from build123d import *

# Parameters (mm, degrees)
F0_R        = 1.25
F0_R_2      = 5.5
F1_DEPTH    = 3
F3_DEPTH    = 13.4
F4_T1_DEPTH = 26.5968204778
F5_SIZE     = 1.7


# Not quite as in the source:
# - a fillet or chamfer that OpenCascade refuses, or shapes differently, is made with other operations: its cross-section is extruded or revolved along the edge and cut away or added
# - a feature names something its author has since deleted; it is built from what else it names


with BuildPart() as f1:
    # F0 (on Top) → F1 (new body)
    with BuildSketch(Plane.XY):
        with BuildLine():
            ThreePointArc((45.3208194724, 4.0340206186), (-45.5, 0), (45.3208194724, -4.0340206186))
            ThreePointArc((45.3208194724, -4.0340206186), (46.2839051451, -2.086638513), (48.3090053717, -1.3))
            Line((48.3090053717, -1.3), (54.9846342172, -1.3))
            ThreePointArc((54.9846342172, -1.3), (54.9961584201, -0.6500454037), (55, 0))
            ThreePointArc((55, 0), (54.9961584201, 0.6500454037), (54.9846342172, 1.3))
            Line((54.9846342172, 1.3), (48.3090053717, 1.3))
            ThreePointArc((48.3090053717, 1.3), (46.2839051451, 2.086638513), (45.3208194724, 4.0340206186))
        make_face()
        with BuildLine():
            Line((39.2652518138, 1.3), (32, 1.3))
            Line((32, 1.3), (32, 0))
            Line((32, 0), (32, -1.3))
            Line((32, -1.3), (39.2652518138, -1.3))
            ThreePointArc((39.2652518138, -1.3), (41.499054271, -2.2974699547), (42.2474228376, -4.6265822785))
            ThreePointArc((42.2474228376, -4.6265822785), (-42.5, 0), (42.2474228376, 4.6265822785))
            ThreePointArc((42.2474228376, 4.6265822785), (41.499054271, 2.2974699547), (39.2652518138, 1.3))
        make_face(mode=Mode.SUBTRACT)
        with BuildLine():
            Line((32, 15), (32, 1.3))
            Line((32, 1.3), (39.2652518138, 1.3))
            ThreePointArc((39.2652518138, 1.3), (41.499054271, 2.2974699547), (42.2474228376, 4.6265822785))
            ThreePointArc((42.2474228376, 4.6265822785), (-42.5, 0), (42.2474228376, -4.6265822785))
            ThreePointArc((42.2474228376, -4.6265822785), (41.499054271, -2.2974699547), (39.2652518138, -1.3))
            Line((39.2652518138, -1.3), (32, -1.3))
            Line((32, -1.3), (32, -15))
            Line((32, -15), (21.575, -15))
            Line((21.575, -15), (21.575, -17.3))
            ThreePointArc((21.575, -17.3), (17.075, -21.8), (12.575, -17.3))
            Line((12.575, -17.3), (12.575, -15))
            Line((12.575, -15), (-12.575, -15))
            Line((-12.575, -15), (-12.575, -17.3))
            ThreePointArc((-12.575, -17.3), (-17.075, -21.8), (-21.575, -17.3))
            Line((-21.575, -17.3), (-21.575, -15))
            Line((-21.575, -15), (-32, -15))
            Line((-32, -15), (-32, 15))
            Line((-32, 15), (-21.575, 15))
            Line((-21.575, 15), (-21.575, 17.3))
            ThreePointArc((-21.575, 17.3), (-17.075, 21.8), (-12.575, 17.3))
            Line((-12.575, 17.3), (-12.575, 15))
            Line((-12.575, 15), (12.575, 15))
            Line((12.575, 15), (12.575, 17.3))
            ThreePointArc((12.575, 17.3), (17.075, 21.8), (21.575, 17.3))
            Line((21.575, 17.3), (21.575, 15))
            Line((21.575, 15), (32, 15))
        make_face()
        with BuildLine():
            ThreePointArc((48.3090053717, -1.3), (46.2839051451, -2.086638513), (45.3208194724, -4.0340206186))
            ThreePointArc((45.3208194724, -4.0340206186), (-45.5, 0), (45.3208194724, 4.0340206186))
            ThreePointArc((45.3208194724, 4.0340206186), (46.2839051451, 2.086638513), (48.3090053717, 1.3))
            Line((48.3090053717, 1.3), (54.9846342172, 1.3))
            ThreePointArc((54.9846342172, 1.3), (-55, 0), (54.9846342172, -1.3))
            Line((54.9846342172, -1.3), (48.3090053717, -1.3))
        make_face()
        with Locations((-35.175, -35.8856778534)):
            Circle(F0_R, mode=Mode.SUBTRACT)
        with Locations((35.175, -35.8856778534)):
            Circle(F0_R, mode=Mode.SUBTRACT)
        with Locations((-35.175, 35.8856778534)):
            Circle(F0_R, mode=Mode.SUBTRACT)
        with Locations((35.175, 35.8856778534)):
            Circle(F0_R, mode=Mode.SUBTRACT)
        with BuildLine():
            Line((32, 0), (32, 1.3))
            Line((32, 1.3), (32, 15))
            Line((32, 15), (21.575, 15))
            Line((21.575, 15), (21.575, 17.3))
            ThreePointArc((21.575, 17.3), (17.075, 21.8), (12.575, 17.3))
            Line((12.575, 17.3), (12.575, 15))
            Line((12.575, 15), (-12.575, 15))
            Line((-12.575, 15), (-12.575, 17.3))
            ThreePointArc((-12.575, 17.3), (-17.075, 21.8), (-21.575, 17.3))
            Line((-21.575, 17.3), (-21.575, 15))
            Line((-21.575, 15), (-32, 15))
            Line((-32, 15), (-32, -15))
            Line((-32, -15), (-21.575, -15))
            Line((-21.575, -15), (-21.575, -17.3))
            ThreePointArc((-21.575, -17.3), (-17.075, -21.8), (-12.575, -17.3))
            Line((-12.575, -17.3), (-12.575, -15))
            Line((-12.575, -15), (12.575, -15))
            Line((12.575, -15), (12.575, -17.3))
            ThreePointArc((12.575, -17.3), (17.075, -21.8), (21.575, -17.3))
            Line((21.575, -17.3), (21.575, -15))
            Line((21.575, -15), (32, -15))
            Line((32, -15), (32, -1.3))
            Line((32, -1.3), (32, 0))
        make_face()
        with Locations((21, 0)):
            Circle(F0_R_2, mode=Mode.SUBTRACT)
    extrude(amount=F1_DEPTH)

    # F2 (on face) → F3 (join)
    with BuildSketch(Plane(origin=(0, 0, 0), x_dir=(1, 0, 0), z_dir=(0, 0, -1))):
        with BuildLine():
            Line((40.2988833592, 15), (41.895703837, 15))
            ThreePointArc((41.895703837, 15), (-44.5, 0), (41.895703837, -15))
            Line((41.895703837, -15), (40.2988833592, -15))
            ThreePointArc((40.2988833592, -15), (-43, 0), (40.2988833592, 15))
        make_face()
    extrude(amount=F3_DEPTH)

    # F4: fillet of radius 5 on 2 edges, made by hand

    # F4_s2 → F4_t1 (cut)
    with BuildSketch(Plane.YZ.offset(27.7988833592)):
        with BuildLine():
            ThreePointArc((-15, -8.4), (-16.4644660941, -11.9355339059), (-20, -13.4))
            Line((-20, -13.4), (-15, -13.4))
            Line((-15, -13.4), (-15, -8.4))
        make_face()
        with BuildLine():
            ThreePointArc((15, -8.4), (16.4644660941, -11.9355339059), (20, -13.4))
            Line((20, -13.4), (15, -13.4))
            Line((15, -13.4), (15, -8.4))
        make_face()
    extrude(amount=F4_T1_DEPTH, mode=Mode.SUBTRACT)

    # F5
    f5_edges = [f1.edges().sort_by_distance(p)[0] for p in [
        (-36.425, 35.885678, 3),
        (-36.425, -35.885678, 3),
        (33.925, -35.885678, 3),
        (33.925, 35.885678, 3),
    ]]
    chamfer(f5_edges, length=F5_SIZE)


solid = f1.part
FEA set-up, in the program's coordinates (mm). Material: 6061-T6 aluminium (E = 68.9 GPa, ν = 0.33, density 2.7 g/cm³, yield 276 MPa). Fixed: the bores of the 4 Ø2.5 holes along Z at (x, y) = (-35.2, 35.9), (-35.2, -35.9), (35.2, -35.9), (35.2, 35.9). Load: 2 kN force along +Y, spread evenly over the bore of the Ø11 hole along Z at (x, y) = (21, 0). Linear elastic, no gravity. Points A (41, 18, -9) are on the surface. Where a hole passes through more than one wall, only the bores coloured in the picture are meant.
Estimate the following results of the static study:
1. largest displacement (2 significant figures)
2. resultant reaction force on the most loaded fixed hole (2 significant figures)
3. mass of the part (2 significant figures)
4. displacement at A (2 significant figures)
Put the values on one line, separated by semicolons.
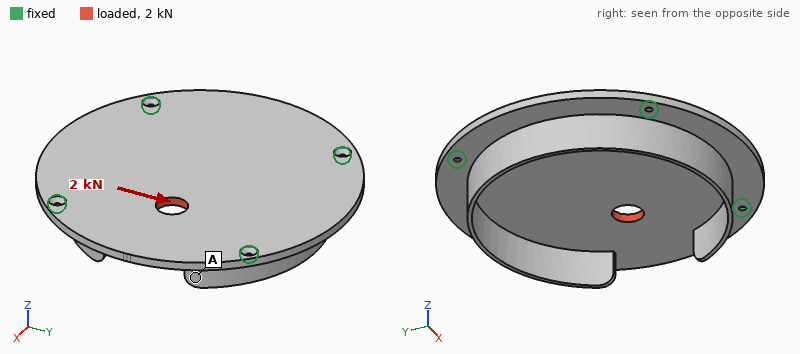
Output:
9.6 µm; 720 N; 89 g; 5.8 µm
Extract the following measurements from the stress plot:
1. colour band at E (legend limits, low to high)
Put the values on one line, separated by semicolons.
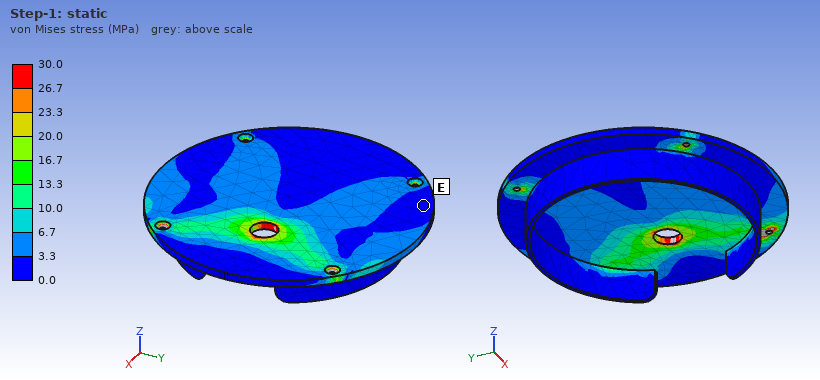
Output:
0.0 to 3.3 MPa
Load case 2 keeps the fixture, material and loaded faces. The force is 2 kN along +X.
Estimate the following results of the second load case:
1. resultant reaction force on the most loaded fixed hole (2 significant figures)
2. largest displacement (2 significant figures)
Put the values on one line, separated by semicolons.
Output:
550 N; 12 µm
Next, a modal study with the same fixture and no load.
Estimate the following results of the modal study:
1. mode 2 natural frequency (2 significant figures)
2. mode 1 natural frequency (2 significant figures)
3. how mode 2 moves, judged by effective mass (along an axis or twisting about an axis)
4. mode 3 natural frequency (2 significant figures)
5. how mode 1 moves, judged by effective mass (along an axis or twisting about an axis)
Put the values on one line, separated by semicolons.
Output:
2300 Hz; 1900 Hz; along Z; 2800 Hz; along Z
